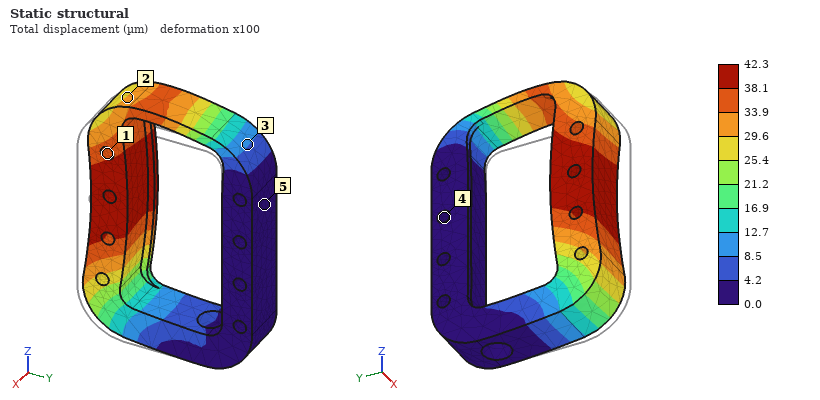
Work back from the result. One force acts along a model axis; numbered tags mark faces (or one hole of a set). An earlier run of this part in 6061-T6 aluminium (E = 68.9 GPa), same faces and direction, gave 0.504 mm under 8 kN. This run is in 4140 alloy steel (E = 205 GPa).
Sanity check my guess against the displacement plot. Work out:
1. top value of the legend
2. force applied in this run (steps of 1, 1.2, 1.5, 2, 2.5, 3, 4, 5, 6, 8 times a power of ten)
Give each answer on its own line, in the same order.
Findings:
42.3 µm
2 kN
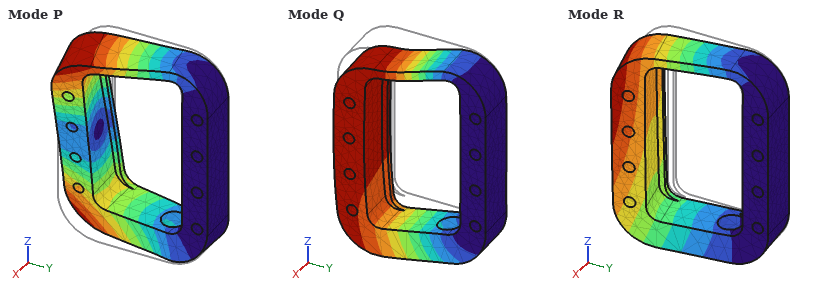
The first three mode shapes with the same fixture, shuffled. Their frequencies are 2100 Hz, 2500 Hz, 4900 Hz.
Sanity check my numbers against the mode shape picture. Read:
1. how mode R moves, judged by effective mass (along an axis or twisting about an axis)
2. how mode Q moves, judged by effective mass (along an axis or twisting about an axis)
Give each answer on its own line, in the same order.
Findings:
along X
along Z
